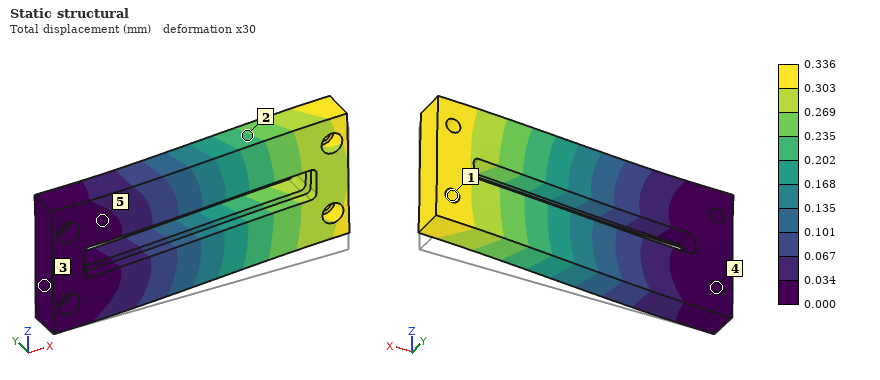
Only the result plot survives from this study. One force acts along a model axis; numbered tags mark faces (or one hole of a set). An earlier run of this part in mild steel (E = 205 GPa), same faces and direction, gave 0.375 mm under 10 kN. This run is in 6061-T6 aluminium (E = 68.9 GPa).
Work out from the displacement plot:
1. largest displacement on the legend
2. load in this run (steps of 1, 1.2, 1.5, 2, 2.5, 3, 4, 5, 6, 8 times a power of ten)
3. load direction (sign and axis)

0.336 mm
3 kN
+Z
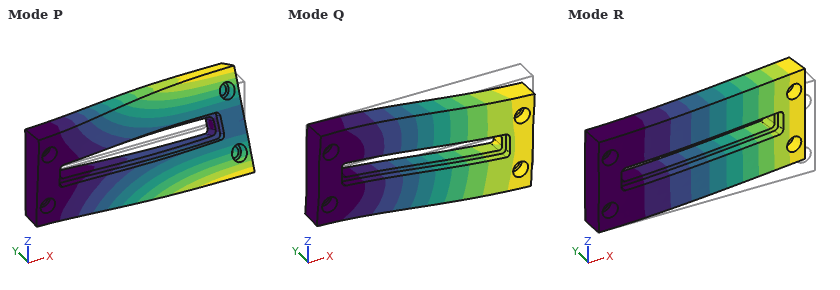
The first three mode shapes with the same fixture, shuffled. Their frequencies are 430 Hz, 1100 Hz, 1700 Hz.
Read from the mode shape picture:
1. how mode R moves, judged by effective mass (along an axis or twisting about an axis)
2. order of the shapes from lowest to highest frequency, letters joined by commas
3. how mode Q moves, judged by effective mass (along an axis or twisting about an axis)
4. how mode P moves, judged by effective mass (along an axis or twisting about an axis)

along Y
R, Q, P
along Z
twisting about X
